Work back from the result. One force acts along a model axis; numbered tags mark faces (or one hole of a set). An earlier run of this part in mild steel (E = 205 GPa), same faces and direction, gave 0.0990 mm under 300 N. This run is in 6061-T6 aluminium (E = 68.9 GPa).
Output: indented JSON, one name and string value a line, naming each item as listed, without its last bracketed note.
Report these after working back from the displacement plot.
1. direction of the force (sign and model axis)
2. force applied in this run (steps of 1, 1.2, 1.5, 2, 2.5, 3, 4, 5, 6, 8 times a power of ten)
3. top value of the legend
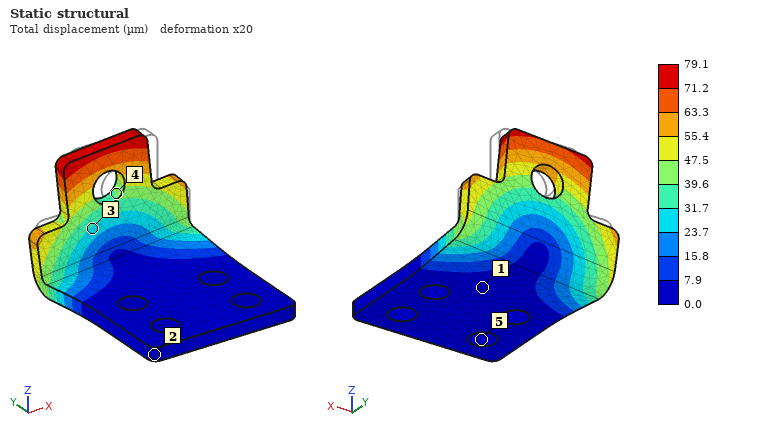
{
  "direction of the force": "-X",
  "force applied in this run": "80 N",
  "top value of the legend": "79.1 µm"
}
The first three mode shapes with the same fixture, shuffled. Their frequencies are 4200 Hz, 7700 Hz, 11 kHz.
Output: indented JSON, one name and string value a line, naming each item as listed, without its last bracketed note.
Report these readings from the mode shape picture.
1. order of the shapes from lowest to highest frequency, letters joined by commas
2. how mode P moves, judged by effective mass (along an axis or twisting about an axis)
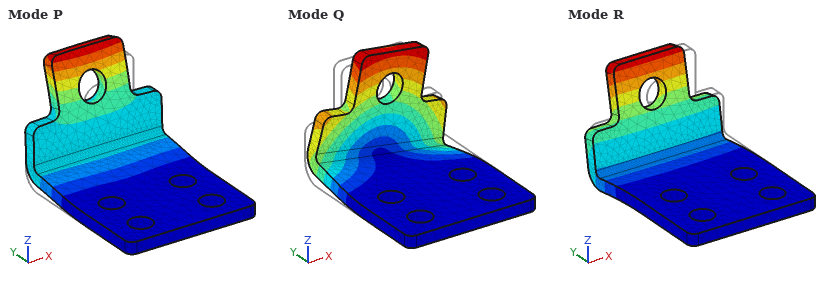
{
  "order of the shapes from lowest to highest frequency, letters joined by commas": "R, Q, P",
  "how mode P moves, judged by effective mass": "along Z"
}
